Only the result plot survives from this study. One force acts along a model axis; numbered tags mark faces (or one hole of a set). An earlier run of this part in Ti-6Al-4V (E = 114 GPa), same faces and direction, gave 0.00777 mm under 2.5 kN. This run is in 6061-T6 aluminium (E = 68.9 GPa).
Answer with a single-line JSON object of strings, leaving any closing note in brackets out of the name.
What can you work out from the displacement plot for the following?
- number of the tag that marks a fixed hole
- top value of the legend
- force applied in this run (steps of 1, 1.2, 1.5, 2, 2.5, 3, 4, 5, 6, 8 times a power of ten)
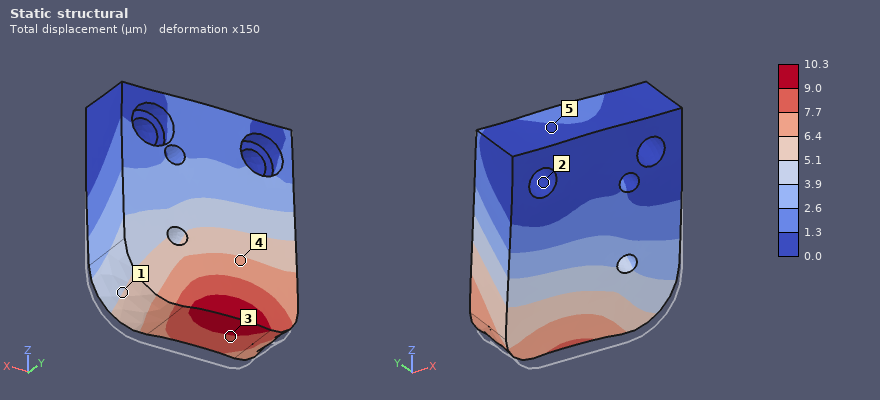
{"number of the tag that marks a fixed hole": "2", "top value of the legend": "10.3 µm", "force applied in this run": "2 kN"}
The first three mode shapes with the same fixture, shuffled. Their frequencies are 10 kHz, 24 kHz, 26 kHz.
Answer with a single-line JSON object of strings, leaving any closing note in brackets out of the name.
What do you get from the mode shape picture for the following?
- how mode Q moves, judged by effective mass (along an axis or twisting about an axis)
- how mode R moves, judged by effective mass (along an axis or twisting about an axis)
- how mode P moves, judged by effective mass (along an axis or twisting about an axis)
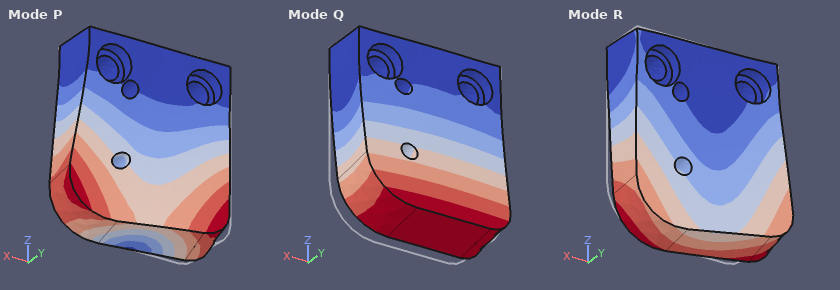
{"how mode Q moves, judged by effective mass": "along Y", "how mode R moves, judged by effective mass": "along X", "how mode P moves, judged by effective mass": "along X"}
